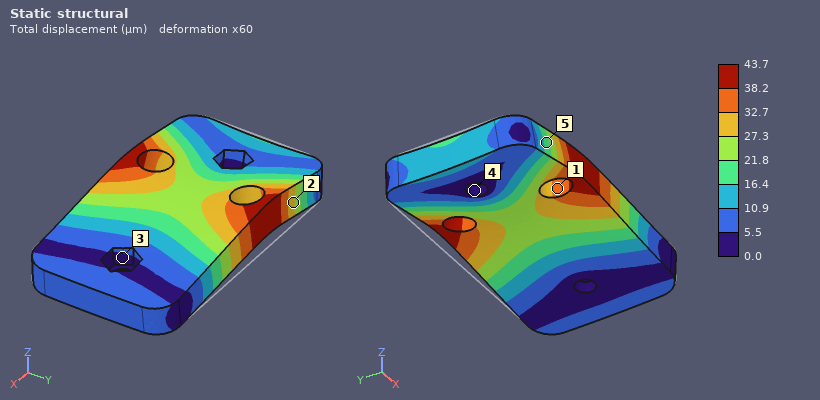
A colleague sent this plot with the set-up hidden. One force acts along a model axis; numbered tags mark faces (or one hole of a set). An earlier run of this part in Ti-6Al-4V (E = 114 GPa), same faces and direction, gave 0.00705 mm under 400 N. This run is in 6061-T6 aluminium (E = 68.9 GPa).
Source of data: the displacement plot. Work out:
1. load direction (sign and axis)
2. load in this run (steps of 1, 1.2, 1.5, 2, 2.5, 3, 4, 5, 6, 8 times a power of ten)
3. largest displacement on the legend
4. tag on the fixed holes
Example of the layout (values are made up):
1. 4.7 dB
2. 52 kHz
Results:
1. +Z
2. 1.5 kN
3. 43.7 µm
4. 4
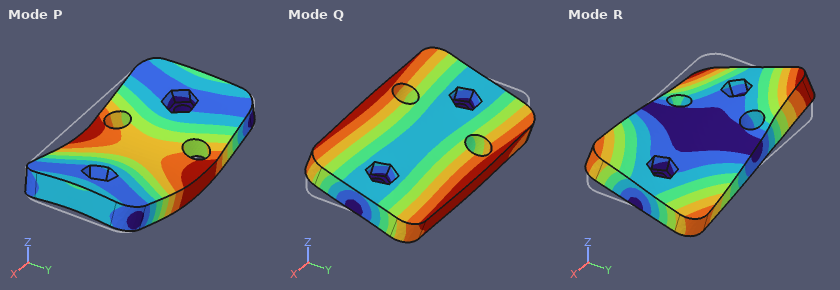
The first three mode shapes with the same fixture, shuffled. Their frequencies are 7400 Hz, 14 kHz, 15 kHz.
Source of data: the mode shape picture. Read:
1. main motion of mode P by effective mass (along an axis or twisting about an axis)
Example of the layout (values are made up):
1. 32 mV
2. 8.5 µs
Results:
1. along Z
